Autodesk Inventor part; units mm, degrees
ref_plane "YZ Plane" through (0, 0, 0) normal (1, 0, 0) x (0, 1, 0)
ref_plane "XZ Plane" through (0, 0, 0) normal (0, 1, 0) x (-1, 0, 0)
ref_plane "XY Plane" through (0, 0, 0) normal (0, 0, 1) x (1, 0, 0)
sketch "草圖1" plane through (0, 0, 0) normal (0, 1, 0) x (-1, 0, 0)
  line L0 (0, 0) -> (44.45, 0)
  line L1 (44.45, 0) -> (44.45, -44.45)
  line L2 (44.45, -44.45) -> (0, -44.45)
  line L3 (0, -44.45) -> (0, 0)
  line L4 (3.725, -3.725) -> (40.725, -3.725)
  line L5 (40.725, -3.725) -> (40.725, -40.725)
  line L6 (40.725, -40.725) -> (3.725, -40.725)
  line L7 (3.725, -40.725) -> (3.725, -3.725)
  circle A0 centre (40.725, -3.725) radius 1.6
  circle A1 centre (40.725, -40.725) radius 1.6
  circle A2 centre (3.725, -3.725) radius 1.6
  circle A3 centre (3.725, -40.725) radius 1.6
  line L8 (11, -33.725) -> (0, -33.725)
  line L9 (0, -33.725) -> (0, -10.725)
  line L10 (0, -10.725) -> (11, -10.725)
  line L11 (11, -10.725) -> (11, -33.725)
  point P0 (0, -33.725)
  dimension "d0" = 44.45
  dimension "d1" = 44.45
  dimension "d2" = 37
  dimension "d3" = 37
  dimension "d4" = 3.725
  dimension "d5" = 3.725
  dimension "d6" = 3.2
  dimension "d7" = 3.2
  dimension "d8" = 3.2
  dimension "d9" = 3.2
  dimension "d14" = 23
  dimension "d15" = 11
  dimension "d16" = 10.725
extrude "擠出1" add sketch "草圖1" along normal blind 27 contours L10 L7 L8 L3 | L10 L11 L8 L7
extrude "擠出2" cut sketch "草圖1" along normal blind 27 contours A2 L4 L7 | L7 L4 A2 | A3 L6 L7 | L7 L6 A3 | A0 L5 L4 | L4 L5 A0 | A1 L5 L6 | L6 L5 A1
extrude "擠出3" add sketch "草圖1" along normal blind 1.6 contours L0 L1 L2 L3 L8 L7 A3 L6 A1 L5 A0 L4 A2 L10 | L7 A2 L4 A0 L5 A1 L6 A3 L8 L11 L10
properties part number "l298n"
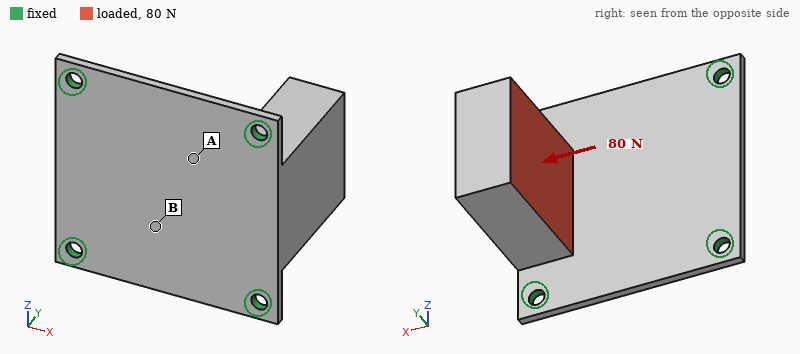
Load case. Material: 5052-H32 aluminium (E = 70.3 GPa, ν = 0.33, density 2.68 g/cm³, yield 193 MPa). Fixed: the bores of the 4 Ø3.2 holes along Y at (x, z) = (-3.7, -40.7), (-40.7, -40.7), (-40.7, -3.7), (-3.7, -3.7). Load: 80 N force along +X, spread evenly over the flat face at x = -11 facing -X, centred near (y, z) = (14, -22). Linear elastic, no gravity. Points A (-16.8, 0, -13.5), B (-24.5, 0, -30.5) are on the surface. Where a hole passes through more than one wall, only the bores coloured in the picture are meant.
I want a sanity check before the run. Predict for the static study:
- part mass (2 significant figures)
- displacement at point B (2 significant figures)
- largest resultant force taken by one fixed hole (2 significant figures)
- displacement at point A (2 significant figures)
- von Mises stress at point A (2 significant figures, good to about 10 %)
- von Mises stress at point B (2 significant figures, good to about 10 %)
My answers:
26 g
22 µm
33 N
24 µm
15 MPa
7.0 MPa
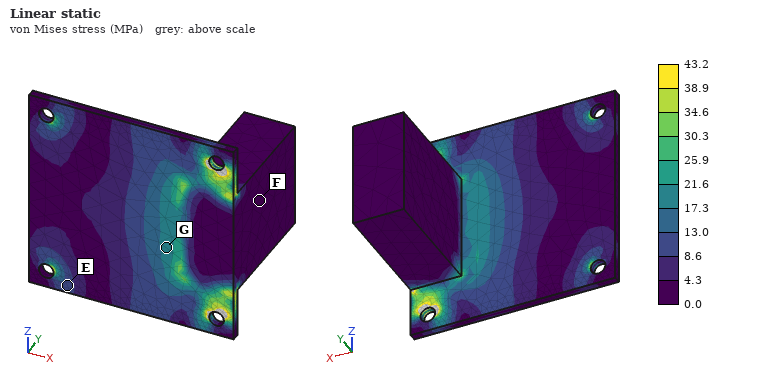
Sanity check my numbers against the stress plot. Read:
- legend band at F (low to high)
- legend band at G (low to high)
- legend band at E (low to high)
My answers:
0.0 to 4.3 MPa
17.3 to 21.6 MPa
8.6 to 13.0 MPa
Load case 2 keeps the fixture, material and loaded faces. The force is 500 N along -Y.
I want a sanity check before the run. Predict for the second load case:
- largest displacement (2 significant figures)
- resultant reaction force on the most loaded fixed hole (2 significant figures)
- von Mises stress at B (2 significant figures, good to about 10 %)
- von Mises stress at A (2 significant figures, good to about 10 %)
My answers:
0.22 mm
230 N
24 MPa
52 MPa
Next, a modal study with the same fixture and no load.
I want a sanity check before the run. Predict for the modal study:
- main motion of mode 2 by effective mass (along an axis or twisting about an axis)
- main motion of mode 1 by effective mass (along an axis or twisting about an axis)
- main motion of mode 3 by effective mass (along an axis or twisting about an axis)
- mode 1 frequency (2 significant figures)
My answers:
along Z
along X
along Y
1400 Hz
